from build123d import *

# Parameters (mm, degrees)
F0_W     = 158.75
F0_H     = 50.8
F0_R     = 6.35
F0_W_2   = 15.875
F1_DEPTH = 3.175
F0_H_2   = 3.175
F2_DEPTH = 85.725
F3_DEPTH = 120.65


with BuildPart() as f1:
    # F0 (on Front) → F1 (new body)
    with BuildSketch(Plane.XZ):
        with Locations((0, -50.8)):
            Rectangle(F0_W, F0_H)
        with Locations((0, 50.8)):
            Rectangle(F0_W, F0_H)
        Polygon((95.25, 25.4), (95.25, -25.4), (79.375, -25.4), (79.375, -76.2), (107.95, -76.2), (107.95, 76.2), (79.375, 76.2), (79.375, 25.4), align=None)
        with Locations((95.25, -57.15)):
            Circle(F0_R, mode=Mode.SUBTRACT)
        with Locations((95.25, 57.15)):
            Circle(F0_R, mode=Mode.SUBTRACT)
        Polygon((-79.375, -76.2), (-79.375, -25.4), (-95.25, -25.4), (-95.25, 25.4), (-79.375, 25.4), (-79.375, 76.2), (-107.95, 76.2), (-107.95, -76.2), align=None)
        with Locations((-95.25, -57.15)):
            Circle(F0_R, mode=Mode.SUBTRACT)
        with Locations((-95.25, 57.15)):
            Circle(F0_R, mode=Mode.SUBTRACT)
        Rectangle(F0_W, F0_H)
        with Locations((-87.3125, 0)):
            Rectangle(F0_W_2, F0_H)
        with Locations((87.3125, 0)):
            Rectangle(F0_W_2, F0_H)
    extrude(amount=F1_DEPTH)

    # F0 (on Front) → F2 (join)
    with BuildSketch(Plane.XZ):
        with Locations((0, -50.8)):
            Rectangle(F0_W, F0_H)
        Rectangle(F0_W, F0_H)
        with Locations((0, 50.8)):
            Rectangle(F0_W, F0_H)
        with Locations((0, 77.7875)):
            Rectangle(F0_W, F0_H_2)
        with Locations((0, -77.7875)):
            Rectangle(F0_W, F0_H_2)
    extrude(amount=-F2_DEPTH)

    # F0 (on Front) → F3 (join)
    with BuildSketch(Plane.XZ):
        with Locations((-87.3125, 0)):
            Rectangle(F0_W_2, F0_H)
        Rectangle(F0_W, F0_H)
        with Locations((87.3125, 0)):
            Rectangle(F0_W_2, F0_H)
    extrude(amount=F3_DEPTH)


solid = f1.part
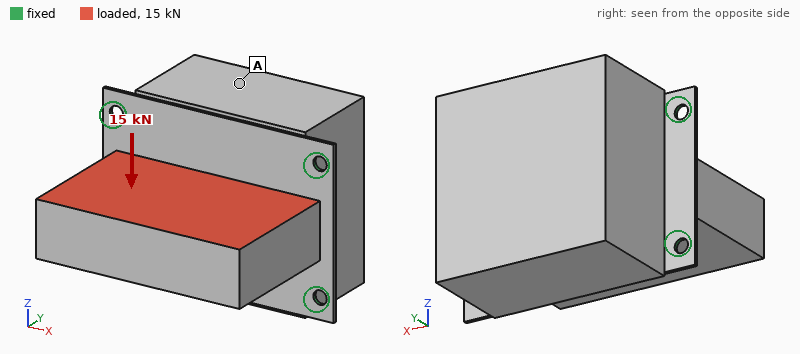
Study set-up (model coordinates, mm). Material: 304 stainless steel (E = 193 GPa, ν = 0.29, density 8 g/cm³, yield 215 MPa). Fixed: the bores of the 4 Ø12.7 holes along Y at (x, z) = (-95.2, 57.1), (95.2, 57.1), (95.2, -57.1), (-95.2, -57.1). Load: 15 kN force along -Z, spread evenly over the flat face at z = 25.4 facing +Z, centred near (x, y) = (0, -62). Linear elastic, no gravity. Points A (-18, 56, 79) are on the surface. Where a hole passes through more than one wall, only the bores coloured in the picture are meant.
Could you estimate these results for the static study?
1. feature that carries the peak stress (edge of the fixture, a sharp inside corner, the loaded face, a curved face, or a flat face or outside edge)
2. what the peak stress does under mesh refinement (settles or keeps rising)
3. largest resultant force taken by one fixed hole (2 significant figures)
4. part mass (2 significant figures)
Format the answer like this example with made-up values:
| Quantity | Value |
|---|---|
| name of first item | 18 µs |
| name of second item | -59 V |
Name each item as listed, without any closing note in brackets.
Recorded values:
| Quantity | Value |
|---|---|
| feature that carries the peak stress | edge of the fixture |
| what the peak stress does under mesh refinement | keeps rising |
| largest resultant force taken by one fixed hole | 5.6 kN |
| part mass | 27 kg |
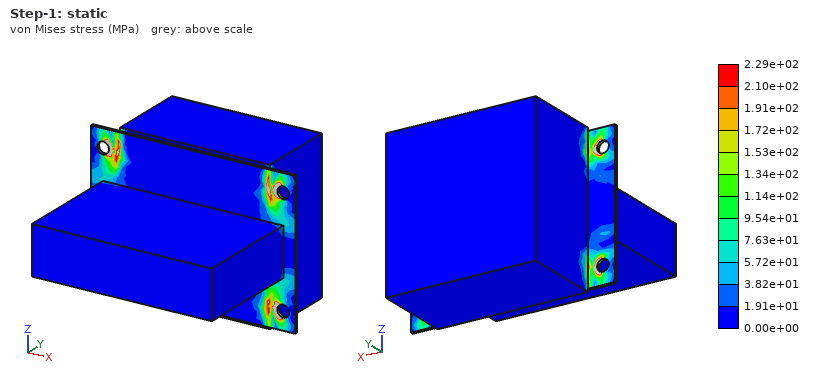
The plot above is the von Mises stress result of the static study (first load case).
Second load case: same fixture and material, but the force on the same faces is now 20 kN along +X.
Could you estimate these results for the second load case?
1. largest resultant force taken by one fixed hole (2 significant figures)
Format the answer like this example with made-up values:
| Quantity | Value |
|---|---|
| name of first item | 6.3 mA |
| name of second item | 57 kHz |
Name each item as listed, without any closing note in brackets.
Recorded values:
| Quantity | Value |
|---|---|
| largest resultant force taken by one fixed hole | 6.5 kN |
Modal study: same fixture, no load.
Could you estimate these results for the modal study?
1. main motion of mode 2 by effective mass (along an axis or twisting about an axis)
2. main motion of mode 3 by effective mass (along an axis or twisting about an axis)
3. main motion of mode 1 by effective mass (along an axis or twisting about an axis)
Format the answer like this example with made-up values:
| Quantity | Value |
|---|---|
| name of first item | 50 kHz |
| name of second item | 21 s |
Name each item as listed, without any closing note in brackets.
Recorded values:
| Quantity | Value |
|---|---|
| main motion of mode 2 by effective mass | along Y |
| main motion of mode 3 by effective mass | twisting about Z |
| main motion of mode 1 by effective mass | twisting about X |
